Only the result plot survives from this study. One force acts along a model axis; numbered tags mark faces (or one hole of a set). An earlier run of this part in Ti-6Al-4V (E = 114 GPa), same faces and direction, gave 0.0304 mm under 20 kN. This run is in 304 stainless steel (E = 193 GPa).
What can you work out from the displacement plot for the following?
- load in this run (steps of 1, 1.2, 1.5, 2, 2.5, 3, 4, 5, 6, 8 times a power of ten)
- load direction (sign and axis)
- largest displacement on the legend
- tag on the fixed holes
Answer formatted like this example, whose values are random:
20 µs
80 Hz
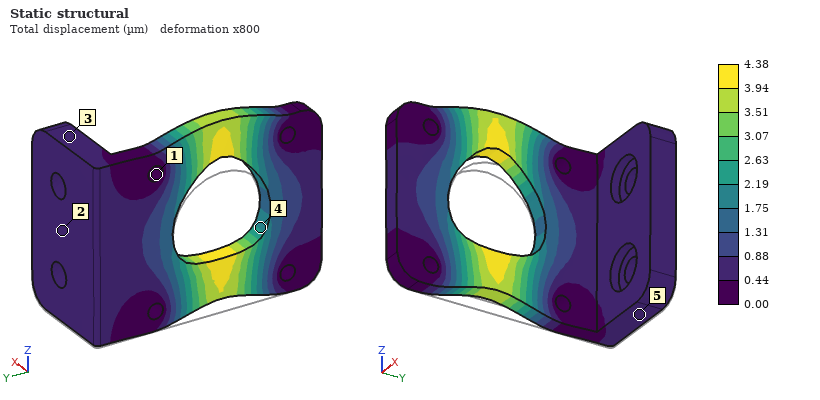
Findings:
5 kN
+Z
4.38 µm
1
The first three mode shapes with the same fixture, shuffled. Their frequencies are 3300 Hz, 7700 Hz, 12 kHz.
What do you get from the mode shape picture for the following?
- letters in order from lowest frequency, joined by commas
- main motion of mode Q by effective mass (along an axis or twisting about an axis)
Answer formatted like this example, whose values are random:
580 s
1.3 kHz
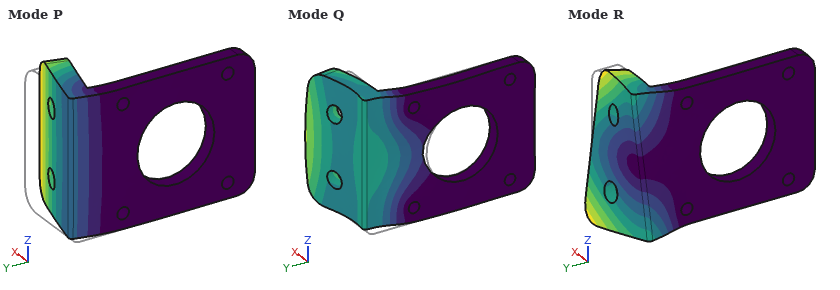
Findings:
P, R, Q
along X
